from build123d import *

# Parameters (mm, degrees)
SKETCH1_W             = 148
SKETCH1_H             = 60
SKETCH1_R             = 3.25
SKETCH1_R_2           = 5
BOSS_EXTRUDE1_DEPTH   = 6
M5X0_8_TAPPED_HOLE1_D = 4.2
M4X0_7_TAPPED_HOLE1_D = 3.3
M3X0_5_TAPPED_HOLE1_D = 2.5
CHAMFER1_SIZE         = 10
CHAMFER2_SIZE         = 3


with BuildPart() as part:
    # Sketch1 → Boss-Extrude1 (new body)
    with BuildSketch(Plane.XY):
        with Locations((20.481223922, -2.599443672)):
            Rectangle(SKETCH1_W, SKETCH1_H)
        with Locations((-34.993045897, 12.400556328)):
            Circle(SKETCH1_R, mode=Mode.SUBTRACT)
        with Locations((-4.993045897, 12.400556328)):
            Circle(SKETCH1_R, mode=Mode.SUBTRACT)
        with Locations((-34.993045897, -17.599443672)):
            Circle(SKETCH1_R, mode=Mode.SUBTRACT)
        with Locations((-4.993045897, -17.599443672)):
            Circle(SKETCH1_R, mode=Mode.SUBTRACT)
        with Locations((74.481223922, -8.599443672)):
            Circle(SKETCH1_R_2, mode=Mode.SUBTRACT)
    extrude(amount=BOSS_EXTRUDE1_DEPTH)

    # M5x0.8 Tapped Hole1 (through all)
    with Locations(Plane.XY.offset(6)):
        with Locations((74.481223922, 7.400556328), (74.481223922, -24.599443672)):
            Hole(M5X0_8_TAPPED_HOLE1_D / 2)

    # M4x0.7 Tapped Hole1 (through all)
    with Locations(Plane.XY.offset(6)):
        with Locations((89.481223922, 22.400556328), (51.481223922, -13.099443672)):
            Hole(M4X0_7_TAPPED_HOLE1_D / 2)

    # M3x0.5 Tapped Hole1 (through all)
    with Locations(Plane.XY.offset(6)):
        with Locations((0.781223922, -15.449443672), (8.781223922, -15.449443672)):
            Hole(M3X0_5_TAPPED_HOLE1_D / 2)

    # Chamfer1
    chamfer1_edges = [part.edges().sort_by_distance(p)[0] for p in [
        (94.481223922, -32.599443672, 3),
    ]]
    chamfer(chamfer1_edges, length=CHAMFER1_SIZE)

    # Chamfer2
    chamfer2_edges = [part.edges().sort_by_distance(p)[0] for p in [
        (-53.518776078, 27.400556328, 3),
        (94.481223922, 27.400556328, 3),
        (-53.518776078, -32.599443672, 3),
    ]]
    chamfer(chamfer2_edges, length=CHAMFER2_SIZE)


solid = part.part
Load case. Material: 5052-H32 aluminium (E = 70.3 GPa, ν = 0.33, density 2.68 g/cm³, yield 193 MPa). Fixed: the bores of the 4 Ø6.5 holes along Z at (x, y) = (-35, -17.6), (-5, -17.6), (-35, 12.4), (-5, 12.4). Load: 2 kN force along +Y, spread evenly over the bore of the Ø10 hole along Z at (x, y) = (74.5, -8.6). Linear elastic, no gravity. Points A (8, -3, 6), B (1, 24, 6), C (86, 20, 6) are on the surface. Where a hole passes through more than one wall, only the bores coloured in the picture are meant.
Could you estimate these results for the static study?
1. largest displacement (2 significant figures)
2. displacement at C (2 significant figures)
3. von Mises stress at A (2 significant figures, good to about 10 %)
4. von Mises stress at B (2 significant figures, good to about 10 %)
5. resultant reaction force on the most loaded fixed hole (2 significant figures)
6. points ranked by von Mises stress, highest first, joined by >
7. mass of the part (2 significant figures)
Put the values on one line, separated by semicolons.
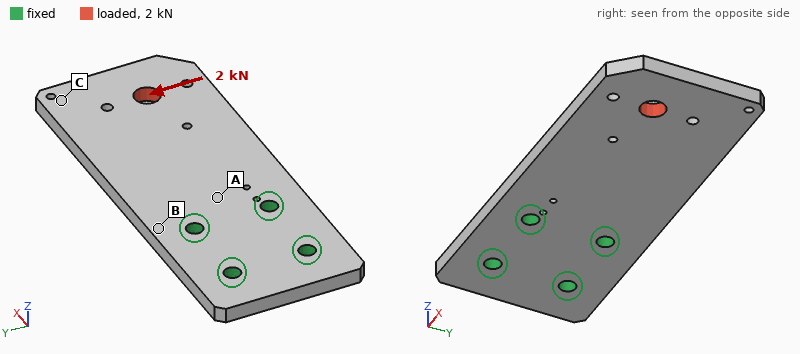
0.10 mm; 0.091 mm; 18 MPa; 28 MPa; 3.6 kN; B > A > C; 140 g
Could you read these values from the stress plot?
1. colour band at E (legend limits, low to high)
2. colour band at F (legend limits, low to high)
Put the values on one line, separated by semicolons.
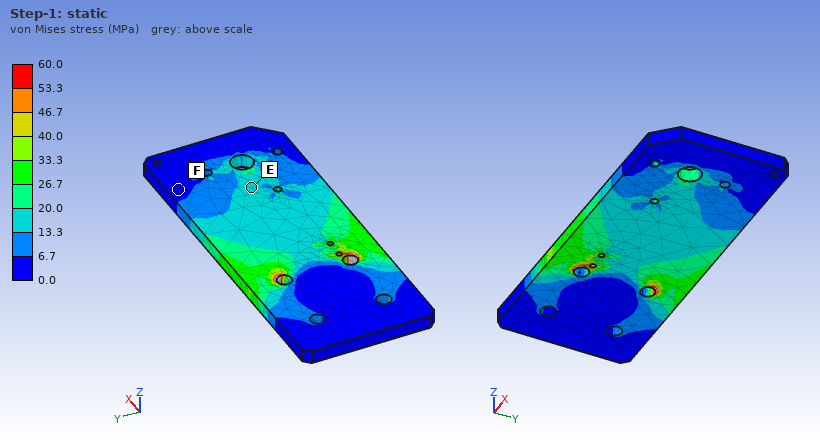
13.3 to 20.0 MPa; 0.0 to 6.7 MPa
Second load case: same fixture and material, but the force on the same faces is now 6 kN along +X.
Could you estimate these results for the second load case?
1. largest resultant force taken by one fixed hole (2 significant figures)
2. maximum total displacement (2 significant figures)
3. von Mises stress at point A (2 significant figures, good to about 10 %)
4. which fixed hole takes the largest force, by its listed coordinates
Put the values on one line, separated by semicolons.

3.3 kN; 38 µm; 14 MPa; (-5, -17.6)
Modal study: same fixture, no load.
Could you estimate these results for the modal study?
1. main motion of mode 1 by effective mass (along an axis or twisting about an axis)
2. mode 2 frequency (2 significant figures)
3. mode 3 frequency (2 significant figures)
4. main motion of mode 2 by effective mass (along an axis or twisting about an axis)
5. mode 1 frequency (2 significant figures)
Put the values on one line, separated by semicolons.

along Z; 1800 Hz; 3100 Hz; twisting about X; 530 Hz
